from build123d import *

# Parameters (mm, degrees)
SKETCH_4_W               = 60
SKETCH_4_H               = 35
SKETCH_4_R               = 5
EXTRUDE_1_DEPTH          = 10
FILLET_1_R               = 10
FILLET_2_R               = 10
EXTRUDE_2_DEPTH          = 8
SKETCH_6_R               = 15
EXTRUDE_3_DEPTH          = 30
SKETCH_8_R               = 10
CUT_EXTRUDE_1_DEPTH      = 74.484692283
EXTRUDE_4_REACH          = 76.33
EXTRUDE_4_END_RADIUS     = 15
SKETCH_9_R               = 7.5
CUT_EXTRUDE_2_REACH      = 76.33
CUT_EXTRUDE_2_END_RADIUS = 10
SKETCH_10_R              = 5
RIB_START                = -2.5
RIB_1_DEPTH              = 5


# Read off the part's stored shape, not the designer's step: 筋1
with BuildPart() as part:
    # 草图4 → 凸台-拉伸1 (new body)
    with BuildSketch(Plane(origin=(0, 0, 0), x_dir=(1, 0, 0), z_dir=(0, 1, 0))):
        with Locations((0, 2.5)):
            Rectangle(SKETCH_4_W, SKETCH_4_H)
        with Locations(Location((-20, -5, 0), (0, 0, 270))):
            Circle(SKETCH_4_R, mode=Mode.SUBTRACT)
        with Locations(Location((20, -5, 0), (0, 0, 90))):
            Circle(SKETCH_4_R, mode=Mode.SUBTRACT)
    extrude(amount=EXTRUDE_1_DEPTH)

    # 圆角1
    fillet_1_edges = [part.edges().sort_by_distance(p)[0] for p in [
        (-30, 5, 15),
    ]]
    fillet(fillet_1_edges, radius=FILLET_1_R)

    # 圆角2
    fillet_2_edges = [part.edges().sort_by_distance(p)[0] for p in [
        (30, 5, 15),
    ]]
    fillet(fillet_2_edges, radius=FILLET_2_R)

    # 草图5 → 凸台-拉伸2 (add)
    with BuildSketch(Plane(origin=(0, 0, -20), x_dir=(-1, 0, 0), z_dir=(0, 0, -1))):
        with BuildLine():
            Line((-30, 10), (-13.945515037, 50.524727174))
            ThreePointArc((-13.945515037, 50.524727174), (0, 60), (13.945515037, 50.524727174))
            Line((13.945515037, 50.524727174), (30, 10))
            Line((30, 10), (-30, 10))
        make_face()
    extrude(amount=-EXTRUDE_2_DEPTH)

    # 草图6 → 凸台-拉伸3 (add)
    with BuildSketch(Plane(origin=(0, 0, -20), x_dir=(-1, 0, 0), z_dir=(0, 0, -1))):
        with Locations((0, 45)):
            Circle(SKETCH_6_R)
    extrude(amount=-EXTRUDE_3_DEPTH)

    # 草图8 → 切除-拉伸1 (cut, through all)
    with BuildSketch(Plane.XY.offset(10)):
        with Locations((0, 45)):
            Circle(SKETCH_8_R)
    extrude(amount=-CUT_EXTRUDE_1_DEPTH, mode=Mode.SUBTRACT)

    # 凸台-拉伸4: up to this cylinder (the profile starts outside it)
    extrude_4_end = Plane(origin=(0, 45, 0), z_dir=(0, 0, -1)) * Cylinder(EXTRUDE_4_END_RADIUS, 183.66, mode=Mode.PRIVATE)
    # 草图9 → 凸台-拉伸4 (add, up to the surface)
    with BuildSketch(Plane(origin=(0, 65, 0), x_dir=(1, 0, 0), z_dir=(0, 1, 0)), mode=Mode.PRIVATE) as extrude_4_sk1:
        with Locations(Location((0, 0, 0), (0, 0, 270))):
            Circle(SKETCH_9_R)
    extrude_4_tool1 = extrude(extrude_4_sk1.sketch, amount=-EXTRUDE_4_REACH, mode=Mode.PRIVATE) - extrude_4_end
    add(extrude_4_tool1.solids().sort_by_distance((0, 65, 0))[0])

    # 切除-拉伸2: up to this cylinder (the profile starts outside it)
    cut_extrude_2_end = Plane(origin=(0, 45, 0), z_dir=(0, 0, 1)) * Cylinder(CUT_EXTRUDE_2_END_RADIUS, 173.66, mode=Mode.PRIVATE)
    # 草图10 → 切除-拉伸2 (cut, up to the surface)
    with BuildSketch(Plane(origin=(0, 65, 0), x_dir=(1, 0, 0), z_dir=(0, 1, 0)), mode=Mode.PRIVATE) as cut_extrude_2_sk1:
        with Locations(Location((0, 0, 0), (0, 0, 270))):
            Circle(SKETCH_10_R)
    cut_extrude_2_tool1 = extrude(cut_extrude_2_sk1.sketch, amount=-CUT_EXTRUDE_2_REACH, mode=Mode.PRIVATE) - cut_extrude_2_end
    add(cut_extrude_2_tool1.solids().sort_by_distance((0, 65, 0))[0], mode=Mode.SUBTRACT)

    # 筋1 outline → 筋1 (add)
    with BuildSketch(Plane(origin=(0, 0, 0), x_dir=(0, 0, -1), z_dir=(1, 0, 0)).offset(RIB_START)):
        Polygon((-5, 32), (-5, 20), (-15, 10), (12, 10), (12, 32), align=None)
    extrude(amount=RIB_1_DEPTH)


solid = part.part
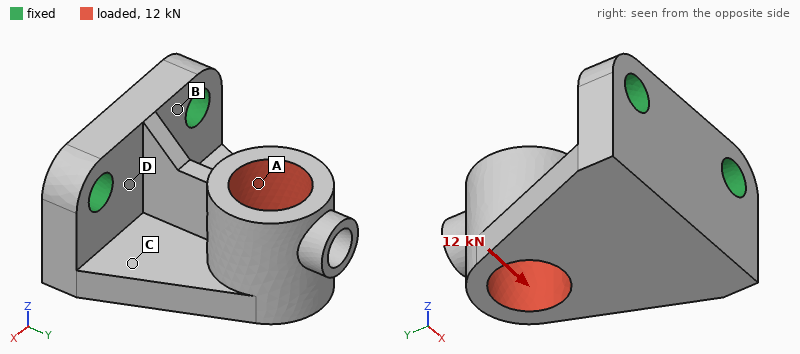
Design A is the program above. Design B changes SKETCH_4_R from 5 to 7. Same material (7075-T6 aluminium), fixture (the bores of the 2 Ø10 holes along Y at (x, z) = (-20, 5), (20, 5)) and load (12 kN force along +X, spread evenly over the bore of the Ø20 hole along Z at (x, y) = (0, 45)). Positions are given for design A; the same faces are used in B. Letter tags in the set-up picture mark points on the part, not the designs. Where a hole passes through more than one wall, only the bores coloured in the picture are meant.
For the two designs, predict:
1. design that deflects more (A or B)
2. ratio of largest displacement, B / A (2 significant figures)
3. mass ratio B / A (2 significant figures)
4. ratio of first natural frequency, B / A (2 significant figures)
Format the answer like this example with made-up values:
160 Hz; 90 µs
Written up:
A; 0.89; 0.96; 1.1
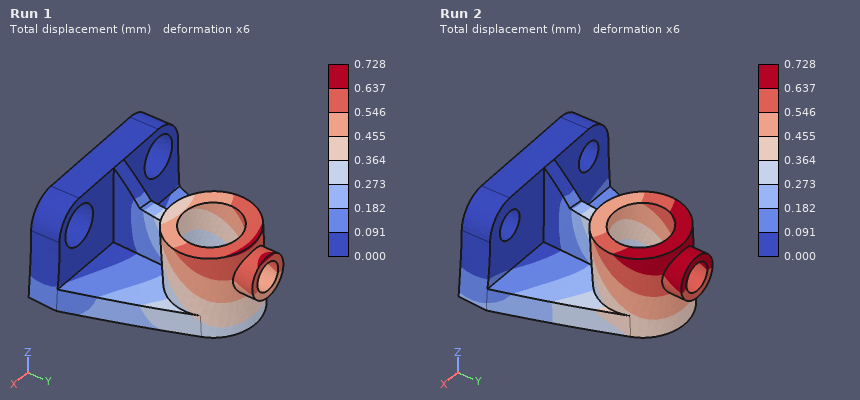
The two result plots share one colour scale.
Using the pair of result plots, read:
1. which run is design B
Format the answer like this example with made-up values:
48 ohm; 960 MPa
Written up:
Run 1
